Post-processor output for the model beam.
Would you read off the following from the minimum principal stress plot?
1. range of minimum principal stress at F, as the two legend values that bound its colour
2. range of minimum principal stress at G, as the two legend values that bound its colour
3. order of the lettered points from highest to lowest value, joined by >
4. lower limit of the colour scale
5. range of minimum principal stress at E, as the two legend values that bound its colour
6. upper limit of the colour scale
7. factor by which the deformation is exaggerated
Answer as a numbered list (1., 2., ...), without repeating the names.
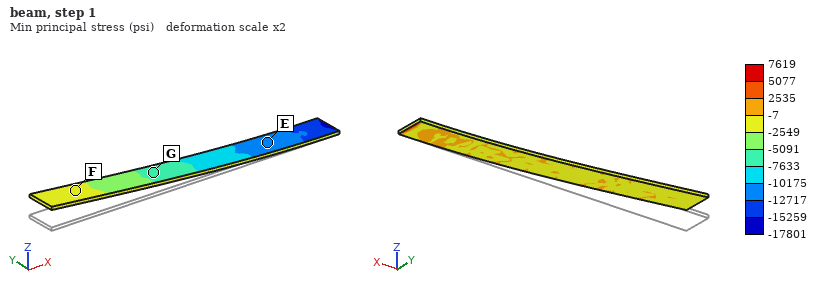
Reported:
1. -2549 to -7 psi
2. -7633 to -5091 psi
3. F > G > E
4. -17801 psi
5. -12717 to -10175 psi
6. 7619 psi
7. 2
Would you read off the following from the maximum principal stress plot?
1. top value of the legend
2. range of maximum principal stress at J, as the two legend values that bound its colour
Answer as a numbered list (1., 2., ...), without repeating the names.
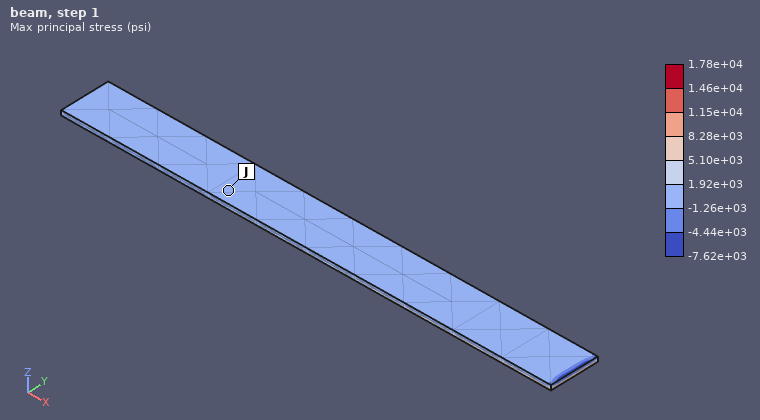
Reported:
1. 1.78e+04 psi
2. -1.26e+03 to 1.92e+03 psi
